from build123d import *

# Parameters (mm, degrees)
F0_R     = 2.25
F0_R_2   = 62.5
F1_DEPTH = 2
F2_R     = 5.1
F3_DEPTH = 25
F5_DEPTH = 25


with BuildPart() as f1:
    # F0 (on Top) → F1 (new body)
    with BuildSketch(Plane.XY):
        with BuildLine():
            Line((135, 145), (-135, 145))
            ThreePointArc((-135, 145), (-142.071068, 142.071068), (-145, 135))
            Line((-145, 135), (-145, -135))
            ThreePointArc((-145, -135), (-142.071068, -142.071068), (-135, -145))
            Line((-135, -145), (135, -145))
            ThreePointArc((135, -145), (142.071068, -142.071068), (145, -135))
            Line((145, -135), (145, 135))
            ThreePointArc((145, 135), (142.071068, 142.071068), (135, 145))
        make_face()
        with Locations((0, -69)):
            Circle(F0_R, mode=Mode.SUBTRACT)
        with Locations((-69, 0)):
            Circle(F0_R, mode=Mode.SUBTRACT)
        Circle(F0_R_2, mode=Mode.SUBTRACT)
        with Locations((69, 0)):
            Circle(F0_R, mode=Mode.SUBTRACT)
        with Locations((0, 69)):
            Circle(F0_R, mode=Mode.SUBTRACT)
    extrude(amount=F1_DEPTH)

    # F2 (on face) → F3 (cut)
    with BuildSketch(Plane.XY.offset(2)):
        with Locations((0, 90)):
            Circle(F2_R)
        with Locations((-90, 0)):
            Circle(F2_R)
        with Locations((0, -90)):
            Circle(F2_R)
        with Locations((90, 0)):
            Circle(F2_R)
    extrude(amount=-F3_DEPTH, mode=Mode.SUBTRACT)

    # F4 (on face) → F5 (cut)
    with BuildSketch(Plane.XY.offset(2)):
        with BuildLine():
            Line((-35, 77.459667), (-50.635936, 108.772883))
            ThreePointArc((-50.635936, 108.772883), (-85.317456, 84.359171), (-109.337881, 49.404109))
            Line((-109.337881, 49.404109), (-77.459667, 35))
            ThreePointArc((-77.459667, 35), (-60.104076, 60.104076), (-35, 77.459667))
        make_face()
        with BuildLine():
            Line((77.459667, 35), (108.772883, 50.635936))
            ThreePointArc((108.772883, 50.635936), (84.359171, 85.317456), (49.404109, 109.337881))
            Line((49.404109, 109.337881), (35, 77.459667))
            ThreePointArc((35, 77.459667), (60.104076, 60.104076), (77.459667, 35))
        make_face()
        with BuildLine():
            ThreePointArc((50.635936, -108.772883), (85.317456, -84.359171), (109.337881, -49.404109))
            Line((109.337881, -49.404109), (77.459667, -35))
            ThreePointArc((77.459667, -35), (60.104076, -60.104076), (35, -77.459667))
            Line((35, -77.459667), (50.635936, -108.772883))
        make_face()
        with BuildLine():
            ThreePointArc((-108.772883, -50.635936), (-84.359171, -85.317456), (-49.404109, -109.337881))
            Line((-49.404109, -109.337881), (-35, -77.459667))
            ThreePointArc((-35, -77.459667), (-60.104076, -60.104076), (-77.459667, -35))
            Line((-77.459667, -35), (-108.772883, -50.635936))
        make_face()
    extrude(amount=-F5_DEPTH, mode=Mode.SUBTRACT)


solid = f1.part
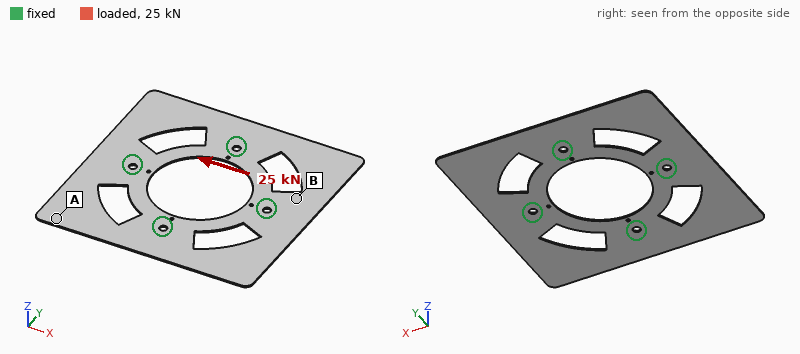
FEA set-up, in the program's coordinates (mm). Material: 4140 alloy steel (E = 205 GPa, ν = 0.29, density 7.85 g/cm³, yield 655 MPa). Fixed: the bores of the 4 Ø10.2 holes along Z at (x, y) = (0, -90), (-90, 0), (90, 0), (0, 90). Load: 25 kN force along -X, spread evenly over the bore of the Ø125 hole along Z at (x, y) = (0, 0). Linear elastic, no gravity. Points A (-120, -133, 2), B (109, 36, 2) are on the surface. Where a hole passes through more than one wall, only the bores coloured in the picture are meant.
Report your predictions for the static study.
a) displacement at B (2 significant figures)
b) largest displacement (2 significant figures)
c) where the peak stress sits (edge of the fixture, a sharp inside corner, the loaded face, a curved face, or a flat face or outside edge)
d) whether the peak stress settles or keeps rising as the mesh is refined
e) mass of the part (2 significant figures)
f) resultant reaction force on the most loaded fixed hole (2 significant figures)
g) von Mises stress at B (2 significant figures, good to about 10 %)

7.3 µm
36 µm
edge of the fixture
keeps rising
960 g
6.9 kN
20 MPa
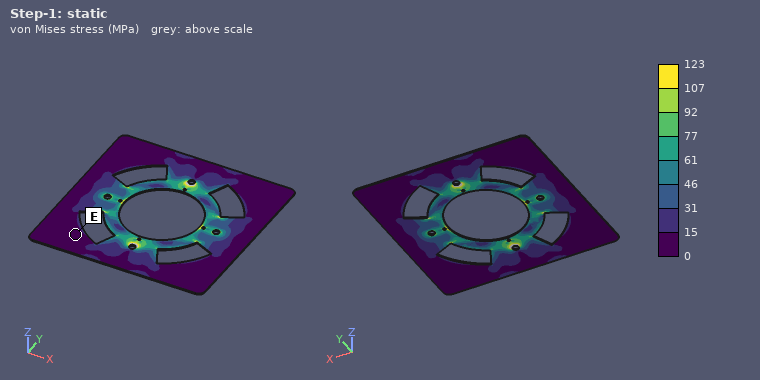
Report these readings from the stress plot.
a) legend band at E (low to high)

0 to 15 MPa
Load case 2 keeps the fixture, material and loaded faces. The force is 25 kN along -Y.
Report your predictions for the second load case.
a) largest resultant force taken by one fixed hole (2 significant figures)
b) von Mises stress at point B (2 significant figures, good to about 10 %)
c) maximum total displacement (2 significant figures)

6.9 kN
19 MPa
36 µm
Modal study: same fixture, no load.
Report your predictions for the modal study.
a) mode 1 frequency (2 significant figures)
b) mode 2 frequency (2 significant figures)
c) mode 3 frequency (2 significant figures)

120 Hz
120 Hz
120 Hz
